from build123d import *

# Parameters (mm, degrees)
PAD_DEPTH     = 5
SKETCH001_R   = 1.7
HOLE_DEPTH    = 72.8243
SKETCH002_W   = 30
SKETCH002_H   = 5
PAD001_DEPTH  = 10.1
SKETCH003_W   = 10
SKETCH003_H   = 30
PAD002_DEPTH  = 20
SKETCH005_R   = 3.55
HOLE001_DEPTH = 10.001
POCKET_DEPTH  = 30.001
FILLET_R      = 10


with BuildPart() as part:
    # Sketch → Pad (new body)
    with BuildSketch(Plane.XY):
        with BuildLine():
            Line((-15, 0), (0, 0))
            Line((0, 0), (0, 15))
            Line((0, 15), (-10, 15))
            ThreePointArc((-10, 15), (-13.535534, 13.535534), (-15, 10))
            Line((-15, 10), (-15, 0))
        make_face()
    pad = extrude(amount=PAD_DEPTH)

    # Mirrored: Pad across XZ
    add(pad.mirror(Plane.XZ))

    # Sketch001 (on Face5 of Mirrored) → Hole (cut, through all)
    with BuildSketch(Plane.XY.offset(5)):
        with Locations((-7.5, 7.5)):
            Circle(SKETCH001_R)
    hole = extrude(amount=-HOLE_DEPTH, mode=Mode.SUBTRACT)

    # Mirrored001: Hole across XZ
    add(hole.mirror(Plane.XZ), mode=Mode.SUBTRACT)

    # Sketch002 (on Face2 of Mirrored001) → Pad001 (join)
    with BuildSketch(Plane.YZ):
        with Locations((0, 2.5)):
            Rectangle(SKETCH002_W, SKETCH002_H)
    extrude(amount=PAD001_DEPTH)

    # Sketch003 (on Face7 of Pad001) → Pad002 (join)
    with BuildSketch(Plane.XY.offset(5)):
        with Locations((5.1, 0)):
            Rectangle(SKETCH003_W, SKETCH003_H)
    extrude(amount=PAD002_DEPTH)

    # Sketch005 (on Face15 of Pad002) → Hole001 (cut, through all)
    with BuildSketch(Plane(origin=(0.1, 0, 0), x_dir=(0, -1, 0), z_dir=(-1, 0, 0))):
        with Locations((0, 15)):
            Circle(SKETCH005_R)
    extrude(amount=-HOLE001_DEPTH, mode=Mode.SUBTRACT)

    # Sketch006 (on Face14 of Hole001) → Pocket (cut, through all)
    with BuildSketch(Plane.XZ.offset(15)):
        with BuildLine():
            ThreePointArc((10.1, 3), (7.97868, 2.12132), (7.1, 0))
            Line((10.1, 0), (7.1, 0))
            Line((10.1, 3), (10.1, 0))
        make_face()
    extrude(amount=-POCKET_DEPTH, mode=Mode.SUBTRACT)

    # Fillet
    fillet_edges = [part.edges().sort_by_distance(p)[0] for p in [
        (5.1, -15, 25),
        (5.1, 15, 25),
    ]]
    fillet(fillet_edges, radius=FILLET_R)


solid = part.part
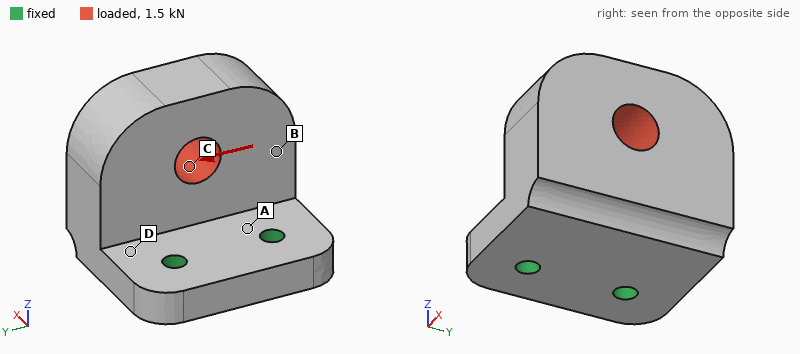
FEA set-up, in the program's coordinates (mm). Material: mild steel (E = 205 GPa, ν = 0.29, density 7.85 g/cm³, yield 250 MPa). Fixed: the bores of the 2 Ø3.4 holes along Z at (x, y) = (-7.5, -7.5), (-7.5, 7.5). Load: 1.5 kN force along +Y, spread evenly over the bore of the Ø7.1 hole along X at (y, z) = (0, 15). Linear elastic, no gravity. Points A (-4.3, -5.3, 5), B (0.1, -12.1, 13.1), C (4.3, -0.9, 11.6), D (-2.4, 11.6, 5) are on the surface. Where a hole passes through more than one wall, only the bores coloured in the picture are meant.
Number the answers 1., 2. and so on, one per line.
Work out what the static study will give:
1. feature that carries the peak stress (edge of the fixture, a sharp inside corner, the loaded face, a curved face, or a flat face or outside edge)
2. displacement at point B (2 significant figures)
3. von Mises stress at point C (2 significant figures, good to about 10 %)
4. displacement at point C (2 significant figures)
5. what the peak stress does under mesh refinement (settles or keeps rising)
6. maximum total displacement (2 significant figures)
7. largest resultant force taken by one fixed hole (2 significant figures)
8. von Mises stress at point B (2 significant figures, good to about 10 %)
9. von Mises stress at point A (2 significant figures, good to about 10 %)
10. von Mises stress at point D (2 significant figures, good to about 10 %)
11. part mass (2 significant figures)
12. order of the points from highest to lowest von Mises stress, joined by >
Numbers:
1. edge of the fixture
2. 12 µm
3. 24 MPa
4. 8.1 µm
5. keeps rising
6. 18 µm
7. 1.6 kN
8. 14 MPa
9. 68 MPa
10. 45 MPa
11. 67 g
12. A > D > C > B
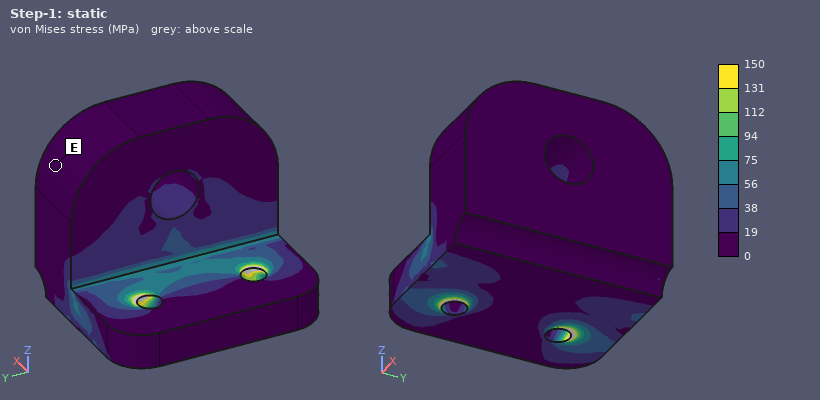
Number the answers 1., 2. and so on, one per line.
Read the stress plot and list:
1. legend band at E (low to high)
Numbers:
1. 0 to 19 MPa
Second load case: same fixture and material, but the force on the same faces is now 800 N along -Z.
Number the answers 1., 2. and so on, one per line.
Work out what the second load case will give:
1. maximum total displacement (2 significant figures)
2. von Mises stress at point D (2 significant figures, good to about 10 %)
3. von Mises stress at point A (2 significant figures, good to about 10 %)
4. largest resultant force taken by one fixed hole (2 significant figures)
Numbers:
1. 27 µm
2. 42 MPa
3. 63 MPa
4. 400 N
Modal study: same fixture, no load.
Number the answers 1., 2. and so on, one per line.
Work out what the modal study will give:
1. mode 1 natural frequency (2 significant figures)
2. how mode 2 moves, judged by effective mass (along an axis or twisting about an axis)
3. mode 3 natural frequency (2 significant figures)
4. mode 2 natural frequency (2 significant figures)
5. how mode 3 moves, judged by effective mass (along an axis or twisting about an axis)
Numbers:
1. 3800 Hz
2. along Y
3. 16 kHz
4. 7800 Hz
5. along Z
